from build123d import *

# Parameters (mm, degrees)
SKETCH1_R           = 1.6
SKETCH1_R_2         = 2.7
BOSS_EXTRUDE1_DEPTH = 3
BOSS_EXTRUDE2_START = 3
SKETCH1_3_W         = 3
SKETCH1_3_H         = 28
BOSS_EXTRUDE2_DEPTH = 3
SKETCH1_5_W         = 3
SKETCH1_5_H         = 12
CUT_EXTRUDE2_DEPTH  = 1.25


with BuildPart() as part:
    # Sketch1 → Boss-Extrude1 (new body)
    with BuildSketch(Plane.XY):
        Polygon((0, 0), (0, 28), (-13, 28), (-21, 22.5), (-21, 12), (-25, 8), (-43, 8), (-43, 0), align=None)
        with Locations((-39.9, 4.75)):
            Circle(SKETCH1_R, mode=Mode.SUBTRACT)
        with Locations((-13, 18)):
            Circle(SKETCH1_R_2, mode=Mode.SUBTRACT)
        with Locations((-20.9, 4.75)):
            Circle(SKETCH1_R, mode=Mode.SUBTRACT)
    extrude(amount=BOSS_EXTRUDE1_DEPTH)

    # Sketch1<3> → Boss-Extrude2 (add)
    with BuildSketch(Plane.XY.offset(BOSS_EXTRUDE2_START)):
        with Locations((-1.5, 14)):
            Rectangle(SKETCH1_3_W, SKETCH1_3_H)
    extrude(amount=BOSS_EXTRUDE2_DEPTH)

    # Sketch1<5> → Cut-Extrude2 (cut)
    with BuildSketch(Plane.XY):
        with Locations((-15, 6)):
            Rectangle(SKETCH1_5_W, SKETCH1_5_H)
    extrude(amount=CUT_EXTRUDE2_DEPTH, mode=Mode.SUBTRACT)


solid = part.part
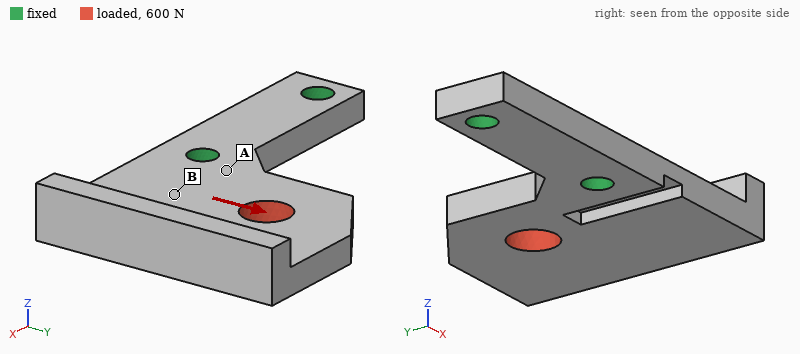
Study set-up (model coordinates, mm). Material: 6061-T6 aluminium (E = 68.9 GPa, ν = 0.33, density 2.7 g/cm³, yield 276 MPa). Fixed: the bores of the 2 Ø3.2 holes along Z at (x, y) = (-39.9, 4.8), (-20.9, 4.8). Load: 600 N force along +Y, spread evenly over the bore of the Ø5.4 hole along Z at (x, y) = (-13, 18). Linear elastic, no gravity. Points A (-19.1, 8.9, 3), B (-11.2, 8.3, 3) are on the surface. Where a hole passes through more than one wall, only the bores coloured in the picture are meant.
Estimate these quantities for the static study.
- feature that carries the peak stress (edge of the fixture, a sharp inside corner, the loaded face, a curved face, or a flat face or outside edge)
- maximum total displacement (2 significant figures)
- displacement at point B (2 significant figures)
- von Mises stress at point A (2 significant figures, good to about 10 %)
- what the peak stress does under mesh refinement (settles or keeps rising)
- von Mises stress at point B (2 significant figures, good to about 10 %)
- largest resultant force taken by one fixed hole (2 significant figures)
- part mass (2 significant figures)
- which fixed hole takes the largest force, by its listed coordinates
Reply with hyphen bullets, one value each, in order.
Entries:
- edge of the fixture
- 75 µm
- 24 µm
- 47 MPa
- keeps rising
- 19 MPa
- 700 N
- 6.3 g
- (-20.9, 4.8)
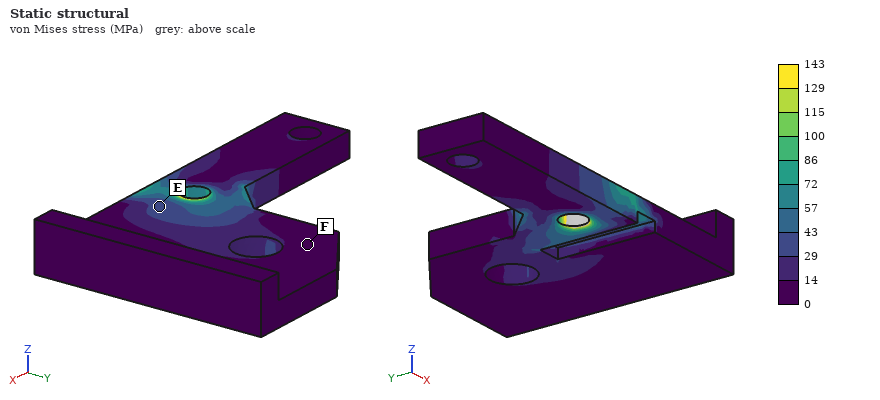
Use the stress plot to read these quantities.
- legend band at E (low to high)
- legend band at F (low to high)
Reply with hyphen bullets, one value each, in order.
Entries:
- 29 to 43 MPa
- 0 to 14 MPa
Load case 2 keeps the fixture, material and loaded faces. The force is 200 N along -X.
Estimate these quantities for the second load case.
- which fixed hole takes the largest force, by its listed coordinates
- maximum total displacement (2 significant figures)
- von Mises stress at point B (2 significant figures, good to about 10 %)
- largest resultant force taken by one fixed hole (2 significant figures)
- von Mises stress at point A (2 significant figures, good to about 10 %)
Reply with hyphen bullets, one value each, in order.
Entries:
- (-20.9, 4.8)
- 42 µm
- 8.6 MPa
- 200 N
- 24 MPa
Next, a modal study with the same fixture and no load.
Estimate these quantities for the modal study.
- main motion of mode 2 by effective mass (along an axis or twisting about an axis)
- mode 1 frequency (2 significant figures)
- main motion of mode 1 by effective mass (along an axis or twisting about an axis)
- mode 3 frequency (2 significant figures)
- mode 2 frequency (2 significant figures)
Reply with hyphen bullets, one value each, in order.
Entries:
- twisting about X
- 2100 Hz
- along Z
- 5600 Hz
- 4600 Hz
